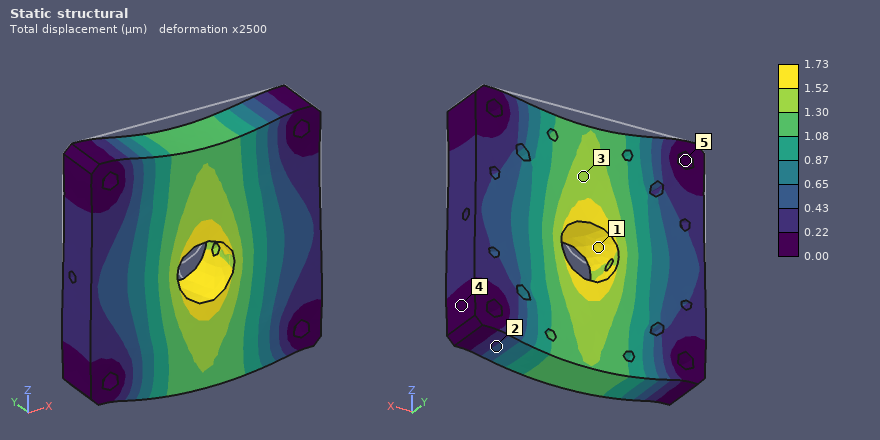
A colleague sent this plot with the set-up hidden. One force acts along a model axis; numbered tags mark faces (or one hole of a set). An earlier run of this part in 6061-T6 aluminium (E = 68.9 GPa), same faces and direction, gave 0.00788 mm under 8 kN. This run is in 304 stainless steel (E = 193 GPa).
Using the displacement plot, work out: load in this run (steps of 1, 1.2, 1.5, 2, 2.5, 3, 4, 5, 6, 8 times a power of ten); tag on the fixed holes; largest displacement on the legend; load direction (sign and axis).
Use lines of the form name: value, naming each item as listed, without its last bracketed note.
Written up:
load in this run: 5 kN
tag on the fixed holes: 5
largest displacement on the legend: 1.73 µm
load direction: -Z
